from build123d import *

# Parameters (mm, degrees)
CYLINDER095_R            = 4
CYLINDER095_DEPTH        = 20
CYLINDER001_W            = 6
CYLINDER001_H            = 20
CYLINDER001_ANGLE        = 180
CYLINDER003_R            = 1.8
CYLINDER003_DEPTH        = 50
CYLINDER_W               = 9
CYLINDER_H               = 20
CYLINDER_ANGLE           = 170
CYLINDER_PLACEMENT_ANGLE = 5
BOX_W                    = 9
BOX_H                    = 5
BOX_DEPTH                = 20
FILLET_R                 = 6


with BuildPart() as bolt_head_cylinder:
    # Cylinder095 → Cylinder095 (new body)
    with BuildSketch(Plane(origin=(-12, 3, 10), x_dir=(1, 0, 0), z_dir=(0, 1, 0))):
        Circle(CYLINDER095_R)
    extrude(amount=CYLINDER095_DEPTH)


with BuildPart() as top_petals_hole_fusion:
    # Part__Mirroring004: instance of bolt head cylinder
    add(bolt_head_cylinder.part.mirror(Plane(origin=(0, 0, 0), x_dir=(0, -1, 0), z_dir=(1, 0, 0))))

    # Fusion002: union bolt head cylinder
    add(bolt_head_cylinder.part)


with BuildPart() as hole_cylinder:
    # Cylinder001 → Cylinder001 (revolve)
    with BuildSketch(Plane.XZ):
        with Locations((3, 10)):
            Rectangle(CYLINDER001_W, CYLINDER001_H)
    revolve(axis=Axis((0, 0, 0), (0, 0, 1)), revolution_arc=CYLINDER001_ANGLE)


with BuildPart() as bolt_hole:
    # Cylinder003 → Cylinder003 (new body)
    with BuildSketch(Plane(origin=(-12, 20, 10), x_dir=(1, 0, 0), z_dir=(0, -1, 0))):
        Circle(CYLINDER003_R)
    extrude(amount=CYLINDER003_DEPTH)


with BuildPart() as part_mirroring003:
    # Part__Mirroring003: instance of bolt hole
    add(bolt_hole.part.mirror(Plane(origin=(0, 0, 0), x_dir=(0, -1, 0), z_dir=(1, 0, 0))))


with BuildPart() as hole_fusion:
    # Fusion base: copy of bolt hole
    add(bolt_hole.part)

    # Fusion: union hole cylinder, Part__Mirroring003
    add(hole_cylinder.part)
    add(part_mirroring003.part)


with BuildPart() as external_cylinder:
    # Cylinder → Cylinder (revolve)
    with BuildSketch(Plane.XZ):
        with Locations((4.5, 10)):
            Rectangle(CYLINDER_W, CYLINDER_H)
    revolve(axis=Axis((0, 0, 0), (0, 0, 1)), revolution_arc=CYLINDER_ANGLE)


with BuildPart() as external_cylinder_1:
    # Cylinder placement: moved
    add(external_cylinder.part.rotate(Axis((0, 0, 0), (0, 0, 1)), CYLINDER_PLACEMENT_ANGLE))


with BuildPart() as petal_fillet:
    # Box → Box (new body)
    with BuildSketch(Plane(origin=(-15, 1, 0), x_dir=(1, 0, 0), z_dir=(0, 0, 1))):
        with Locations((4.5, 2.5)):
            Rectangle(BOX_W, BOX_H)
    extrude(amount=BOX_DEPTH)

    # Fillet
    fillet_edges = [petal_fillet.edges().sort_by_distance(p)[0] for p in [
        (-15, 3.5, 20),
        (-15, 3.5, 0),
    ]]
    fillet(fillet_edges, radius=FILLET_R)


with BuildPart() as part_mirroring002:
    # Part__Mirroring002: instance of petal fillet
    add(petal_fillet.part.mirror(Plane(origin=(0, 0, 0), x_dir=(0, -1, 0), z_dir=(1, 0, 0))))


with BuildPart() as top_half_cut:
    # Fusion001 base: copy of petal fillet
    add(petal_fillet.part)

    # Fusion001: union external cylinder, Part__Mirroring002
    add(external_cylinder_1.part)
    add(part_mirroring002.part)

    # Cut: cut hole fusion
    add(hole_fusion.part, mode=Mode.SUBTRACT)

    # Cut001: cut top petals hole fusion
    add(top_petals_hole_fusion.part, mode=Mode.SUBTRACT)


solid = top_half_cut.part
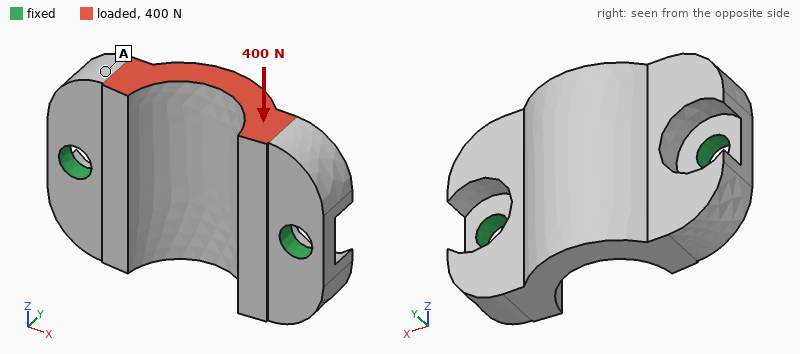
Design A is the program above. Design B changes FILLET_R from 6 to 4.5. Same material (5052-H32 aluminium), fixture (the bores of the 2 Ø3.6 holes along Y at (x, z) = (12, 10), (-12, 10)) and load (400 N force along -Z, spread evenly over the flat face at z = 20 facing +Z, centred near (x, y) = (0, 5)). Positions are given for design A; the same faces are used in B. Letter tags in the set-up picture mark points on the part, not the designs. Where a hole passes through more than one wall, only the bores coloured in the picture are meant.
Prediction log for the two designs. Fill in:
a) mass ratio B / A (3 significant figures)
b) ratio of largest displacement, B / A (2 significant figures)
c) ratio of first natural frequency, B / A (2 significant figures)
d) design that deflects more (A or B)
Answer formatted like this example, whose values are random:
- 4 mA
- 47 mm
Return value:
- 1.03
- 0.91
- 0.98
- A
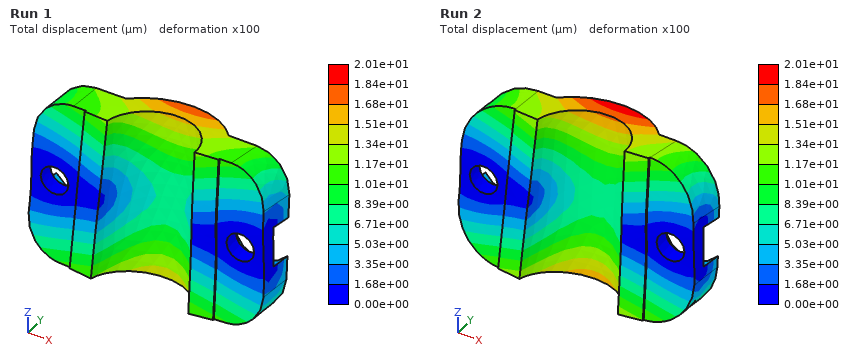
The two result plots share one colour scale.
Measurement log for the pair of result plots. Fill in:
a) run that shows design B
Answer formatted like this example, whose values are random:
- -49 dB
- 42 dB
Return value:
- Run 1
